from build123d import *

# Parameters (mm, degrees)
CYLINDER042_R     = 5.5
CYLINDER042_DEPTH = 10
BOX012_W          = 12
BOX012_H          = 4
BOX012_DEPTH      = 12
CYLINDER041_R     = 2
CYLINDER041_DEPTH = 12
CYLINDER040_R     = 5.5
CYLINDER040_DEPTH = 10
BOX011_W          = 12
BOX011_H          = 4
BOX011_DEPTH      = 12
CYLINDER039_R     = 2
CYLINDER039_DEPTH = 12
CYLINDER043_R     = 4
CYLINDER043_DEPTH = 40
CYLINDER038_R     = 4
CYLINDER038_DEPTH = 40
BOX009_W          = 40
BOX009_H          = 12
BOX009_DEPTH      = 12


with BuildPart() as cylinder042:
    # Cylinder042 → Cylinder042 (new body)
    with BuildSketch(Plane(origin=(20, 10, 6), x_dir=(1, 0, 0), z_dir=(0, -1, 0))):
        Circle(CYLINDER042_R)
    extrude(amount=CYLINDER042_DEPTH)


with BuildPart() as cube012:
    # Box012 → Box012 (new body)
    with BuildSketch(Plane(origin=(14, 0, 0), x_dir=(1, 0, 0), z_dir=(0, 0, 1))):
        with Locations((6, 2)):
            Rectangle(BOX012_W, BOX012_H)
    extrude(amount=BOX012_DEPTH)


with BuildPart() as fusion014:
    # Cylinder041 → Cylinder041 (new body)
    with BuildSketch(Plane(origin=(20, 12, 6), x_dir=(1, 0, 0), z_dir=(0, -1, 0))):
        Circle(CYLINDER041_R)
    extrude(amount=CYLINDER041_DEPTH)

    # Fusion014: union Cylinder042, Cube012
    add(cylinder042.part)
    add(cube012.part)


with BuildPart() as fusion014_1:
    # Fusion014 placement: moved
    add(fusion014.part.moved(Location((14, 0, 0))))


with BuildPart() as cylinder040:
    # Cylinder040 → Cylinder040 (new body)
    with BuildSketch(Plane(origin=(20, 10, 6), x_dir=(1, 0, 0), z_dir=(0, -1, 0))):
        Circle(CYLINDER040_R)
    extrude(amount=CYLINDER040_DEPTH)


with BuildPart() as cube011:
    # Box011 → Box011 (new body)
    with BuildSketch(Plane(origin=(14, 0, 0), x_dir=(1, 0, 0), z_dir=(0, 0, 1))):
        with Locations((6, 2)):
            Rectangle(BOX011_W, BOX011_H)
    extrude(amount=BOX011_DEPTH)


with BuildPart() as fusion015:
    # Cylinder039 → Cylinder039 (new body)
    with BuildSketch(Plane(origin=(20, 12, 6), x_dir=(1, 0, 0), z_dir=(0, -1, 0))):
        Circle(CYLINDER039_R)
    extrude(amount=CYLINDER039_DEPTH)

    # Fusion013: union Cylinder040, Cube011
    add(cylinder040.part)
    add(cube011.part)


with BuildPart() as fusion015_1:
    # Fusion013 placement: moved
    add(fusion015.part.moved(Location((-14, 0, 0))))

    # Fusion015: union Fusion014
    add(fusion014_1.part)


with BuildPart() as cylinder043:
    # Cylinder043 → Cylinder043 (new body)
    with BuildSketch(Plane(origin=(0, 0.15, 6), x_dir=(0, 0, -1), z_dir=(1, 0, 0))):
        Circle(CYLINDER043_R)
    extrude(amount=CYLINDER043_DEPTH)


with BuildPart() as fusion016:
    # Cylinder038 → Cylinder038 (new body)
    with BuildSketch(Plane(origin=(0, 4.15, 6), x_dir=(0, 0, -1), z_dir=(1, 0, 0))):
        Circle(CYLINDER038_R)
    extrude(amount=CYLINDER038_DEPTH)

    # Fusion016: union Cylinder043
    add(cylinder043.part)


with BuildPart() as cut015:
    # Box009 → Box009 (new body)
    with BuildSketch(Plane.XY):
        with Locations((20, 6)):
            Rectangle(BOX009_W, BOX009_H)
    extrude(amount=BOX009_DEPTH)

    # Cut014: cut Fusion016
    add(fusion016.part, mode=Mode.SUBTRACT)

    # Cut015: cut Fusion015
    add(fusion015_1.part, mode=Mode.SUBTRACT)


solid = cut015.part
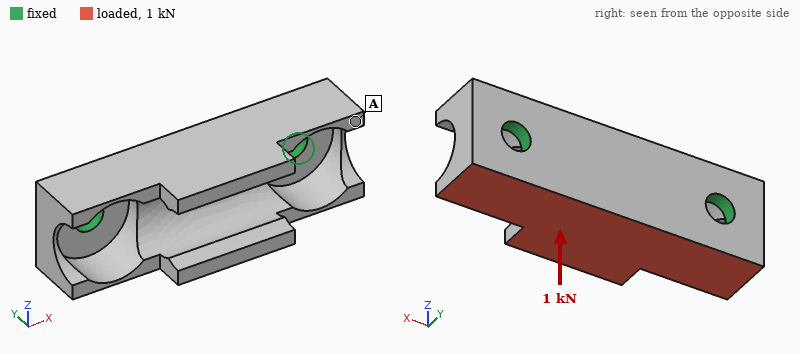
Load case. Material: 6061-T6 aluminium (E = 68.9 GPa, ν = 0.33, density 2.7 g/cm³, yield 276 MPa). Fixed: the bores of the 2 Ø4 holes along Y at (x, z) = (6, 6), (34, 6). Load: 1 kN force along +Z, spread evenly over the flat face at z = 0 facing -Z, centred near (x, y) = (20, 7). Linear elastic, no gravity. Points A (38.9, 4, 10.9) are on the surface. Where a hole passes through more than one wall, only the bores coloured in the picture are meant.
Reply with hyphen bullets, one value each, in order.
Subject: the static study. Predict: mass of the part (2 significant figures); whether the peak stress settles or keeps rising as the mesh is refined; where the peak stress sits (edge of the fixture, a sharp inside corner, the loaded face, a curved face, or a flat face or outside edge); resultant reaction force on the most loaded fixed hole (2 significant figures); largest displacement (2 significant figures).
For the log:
- 6.5 g
- keeps rising
- edge of the fixture
- 500 N
- 70 µm
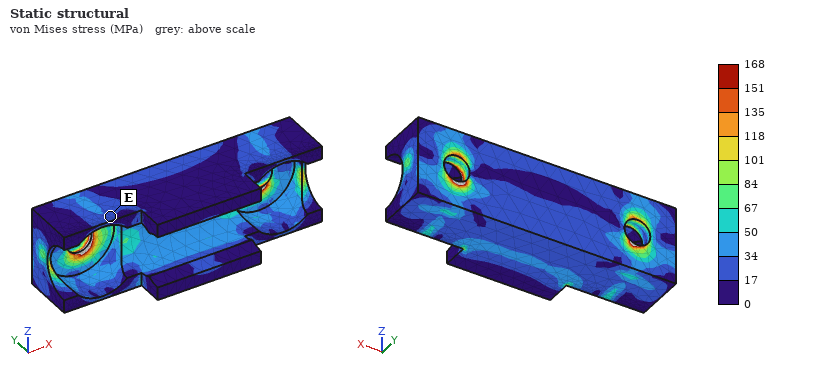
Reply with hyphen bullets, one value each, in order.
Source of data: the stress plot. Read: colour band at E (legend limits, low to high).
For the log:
- 17 to 34 MPa
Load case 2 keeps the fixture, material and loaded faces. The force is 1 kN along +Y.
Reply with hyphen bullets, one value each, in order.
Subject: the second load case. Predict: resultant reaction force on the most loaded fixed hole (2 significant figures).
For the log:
- 530 N
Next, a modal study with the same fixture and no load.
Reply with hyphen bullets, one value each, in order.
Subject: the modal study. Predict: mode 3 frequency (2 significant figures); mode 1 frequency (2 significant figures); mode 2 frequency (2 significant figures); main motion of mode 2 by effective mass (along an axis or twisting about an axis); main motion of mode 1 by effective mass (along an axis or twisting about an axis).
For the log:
- 26 kHz
- 11 kHz
- 21 kHz
- along Y
- along Z
